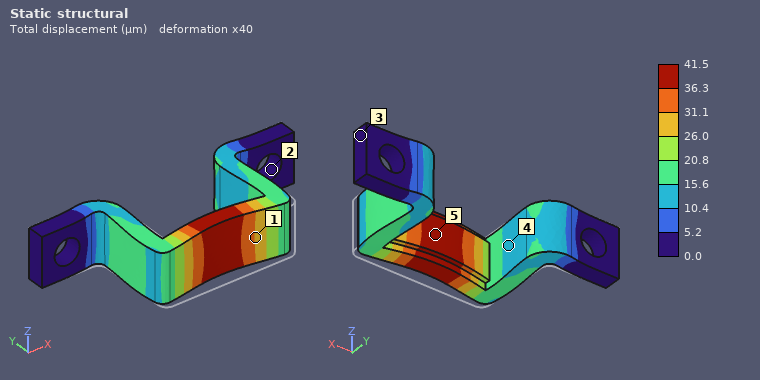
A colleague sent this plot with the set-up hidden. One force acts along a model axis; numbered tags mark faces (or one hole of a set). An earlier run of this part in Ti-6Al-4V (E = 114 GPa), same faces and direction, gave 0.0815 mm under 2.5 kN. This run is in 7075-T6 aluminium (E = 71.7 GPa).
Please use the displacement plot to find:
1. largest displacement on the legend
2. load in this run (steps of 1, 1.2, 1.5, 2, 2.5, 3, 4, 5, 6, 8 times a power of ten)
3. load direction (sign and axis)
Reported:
41.5 µm
800 N
+Y
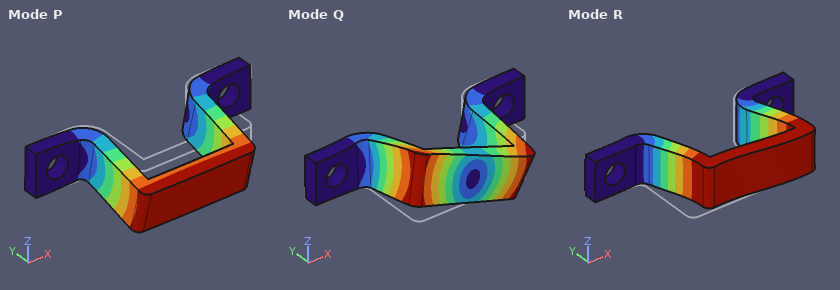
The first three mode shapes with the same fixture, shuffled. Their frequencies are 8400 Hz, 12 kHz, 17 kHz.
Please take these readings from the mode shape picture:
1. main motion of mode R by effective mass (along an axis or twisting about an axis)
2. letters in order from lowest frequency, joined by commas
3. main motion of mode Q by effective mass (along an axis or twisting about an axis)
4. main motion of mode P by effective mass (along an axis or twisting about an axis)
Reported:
along X
P, R, Q
twisting about Y
along Z
